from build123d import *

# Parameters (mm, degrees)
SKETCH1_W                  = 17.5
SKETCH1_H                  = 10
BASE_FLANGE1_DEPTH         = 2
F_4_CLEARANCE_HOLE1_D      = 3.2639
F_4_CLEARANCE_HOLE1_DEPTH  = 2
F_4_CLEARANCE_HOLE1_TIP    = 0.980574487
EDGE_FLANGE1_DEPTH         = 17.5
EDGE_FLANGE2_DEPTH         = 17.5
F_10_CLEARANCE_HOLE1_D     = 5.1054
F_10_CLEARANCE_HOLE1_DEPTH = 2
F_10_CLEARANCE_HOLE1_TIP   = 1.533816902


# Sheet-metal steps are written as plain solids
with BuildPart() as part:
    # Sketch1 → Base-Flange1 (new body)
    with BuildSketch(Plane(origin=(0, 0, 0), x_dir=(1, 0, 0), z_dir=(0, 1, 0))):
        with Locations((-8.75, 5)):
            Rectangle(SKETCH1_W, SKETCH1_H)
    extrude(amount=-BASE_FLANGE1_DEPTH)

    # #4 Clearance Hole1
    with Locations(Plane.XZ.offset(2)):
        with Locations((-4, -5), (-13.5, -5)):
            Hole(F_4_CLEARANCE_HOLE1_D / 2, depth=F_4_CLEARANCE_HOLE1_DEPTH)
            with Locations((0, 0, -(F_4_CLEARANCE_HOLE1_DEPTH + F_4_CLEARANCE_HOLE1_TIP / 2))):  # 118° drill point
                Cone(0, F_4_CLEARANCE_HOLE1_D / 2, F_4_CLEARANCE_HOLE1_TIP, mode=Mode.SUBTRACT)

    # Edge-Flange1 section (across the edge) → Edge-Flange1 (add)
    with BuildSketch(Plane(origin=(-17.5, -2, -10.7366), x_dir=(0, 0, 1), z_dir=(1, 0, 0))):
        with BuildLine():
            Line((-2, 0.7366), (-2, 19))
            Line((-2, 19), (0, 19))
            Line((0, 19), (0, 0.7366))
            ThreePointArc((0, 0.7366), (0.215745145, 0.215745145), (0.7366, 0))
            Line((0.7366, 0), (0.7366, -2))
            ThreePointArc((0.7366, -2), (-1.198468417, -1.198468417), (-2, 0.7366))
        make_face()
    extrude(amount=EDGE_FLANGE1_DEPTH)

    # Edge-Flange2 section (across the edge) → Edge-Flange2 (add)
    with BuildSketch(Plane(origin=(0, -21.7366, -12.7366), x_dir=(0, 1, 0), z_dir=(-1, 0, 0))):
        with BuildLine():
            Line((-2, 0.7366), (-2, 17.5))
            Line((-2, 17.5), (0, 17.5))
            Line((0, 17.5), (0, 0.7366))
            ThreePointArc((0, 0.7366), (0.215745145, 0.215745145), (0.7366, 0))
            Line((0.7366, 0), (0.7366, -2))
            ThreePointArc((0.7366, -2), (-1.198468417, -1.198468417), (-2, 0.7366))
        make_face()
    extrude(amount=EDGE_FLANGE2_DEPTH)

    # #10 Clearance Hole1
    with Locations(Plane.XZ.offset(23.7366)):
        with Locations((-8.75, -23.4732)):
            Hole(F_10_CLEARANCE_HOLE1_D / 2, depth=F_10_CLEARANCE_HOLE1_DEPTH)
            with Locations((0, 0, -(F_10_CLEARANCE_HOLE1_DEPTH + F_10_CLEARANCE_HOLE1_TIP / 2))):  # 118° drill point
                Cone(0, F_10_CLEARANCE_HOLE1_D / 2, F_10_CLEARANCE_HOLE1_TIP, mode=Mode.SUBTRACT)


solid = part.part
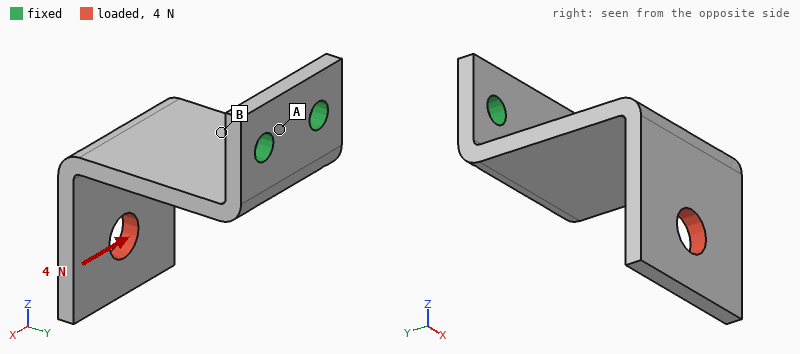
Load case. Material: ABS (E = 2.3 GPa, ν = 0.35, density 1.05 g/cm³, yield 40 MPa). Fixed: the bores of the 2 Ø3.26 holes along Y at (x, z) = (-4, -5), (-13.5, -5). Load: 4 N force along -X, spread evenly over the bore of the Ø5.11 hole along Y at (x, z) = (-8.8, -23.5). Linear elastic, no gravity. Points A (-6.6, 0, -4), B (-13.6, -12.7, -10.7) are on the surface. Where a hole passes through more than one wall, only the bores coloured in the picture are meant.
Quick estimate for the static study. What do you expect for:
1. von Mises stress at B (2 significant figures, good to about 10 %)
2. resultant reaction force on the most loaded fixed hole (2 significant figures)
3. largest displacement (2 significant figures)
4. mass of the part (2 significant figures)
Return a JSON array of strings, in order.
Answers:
["2.9 MPa", "9.9 N", "0.43 mm", "1.8 g"]
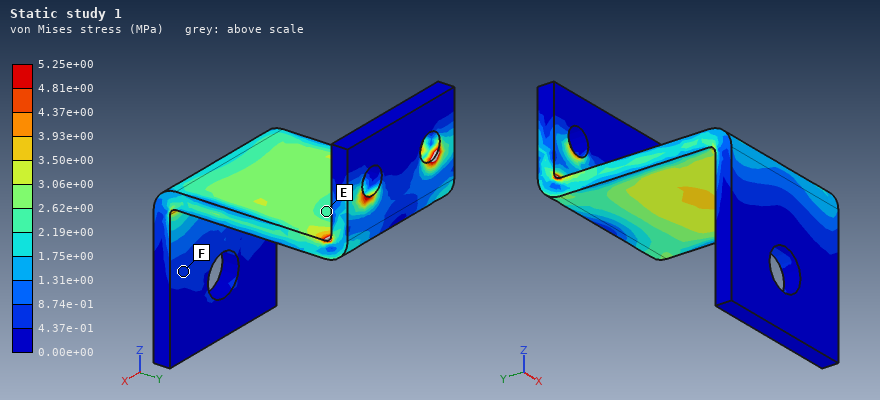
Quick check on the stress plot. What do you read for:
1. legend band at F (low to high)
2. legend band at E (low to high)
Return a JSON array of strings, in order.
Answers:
["4.37e-01 to 8.74e-01 MPa", "2.19e+00 to 2.62e+00 MPa"]
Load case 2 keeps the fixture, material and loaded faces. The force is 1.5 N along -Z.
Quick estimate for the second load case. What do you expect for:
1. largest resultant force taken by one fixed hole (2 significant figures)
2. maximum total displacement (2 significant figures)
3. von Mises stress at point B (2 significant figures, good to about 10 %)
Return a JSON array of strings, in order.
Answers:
["0.95 N", "0.48 mm", "1.2 MPa"]
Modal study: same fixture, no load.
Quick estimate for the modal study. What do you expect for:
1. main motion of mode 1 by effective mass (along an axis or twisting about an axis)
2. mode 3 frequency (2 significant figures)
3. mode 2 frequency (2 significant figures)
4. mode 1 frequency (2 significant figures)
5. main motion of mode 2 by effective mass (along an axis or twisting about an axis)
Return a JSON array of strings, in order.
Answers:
["along Z", "1200 Hz", "760 Hz", "330 Hz", "along X"]
